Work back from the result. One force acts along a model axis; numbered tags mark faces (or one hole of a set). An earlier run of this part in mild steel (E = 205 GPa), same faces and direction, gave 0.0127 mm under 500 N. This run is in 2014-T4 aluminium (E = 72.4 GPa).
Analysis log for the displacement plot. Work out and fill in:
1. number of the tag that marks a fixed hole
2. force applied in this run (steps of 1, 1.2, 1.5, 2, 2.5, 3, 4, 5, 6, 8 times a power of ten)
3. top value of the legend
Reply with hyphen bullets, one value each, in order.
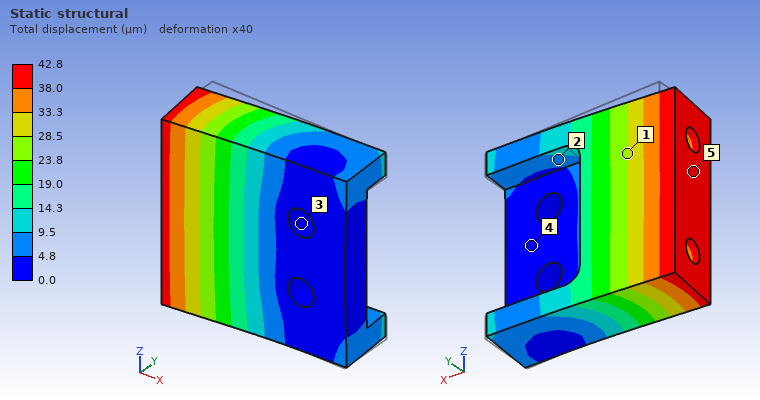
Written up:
- 3
- 600 N
- 42.8 µm
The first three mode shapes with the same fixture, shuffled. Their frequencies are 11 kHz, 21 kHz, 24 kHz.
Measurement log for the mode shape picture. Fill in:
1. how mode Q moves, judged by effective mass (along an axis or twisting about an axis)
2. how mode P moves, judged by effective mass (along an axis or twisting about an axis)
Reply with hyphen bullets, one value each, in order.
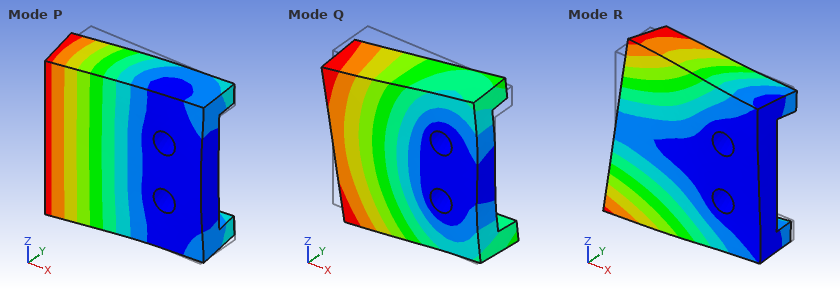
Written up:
- along Z
- along Y
